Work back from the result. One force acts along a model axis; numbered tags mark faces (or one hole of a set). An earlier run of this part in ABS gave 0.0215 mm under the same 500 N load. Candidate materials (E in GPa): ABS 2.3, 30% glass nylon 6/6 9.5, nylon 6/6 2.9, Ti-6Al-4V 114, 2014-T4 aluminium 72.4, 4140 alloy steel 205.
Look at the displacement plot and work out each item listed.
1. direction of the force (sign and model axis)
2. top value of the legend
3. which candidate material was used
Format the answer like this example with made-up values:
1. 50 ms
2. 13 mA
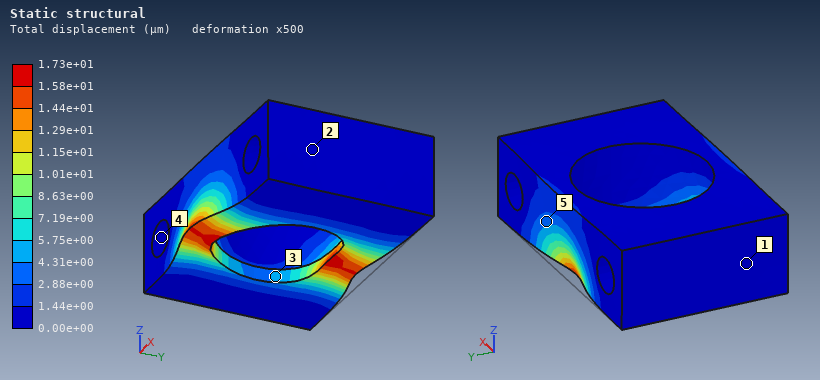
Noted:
1. -Y
2. 1.73e+01 µm
3. nylon 6/6
